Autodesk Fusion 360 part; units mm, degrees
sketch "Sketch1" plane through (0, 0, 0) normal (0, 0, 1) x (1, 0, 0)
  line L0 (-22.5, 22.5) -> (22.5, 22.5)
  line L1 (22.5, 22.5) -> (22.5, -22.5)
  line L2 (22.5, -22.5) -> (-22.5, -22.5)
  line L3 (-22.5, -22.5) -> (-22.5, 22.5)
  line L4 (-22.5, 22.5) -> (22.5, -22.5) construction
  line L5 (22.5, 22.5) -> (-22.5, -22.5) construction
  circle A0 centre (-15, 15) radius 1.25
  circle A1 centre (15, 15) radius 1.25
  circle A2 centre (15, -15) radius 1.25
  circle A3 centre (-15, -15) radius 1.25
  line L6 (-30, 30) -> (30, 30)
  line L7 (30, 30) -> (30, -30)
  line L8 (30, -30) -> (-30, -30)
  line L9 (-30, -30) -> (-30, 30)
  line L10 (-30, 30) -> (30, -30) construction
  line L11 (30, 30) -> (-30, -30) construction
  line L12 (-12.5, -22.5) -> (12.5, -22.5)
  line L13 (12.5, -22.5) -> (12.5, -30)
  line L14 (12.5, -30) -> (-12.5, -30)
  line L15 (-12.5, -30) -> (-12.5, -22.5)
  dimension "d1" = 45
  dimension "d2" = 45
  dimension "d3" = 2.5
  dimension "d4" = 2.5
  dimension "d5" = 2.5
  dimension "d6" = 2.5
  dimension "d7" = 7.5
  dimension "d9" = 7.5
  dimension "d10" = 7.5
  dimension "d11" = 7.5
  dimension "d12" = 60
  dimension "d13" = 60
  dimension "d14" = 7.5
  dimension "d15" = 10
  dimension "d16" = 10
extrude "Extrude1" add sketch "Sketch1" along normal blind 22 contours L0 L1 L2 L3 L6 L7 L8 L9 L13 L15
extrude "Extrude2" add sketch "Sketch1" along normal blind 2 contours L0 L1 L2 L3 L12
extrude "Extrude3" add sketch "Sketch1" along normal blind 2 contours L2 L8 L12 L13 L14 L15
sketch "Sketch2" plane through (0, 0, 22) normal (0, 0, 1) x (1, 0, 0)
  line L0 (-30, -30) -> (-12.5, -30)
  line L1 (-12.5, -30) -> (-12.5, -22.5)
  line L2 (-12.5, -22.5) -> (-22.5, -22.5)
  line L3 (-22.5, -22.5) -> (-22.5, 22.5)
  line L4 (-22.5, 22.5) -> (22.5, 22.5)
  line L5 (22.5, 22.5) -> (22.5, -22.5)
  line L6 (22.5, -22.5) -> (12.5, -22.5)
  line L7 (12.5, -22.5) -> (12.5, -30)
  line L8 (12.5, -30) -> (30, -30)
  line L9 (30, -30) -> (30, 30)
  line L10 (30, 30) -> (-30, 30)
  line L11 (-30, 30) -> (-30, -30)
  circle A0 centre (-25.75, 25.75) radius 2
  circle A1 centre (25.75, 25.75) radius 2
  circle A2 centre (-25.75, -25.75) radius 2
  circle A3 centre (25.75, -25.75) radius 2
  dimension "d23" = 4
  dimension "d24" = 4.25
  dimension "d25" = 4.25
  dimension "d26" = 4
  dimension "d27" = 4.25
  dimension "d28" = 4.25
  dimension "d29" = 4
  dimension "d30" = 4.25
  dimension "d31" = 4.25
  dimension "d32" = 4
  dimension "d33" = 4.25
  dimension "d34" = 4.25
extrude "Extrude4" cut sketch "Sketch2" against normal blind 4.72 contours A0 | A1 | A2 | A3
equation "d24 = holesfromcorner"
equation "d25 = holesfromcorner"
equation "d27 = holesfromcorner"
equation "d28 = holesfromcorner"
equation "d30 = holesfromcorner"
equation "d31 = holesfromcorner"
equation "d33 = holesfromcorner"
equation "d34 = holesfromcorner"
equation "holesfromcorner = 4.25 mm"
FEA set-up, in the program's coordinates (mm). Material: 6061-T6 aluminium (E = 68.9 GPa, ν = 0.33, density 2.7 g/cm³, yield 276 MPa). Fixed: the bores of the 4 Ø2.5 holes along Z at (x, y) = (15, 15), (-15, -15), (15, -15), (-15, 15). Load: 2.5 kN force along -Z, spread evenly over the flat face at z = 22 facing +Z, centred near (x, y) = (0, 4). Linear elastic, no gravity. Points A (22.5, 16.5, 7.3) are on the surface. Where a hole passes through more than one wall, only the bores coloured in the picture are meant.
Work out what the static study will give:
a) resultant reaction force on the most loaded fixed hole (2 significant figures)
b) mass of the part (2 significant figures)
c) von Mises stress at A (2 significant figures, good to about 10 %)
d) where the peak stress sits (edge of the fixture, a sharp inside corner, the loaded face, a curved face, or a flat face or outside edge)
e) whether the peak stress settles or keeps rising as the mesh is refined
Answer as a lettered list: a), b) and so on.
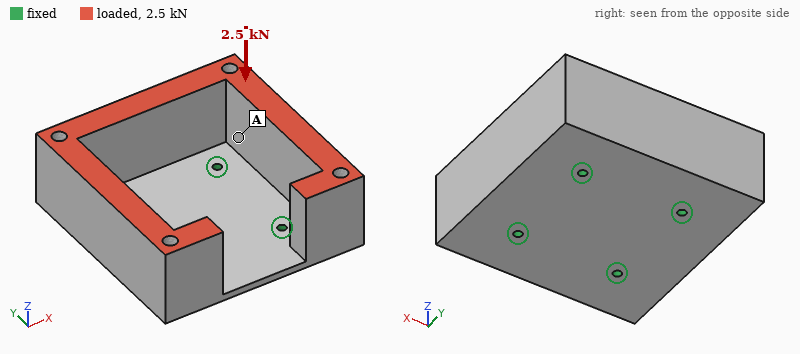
a) 790 N
b) 94 g
c) 17 MPa
d) edge of the fixture
e) keeps rising
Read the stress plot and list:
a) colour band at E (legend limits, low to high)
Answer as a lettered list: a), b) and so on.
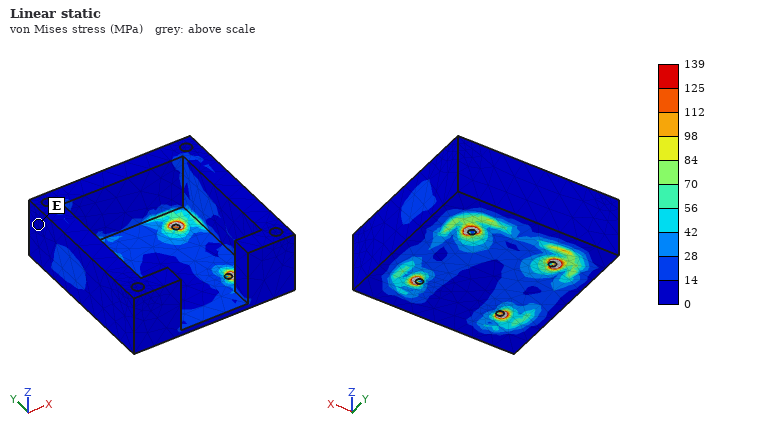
a) 0 to 14 MPa
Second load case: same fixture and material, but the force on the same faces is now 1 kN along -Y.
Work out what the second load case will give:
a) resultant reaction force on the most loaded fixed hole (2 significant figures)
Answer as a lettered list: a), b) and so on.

a) 410 N
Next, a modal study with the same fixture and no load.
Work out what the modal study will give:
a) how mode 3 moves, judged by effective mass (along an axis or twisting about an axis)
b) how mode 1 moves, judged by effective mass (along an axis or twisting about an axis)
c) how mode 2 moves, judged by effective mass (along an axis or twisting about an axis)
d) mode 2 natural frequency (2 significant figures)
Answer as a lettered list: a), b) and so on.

a) along Z
b) along X
c) along Y
d) 2800 Hz
